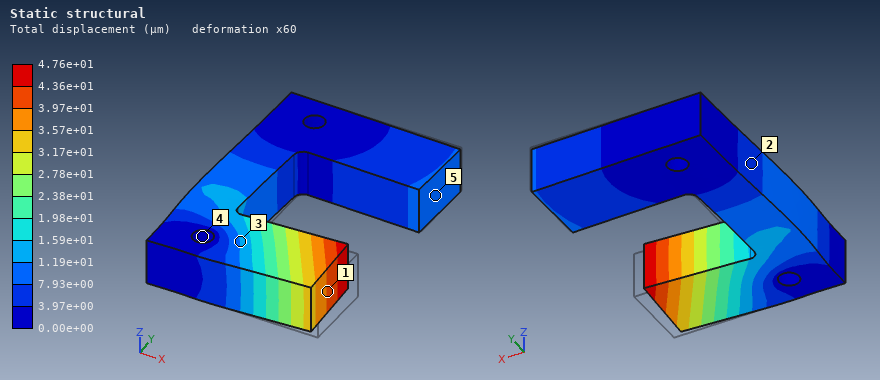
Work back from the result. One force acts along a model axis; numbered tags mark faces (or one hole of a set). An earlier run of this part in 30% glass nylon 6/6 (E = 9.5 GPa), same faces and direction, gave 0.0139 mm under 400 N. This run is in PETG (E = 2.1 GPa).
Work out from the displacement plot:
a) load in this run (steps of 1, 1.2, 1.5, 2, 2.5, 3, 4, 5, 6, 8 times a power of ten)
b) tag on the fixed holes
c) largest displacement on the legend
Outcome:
300 N
4
4.76e+01 µm
